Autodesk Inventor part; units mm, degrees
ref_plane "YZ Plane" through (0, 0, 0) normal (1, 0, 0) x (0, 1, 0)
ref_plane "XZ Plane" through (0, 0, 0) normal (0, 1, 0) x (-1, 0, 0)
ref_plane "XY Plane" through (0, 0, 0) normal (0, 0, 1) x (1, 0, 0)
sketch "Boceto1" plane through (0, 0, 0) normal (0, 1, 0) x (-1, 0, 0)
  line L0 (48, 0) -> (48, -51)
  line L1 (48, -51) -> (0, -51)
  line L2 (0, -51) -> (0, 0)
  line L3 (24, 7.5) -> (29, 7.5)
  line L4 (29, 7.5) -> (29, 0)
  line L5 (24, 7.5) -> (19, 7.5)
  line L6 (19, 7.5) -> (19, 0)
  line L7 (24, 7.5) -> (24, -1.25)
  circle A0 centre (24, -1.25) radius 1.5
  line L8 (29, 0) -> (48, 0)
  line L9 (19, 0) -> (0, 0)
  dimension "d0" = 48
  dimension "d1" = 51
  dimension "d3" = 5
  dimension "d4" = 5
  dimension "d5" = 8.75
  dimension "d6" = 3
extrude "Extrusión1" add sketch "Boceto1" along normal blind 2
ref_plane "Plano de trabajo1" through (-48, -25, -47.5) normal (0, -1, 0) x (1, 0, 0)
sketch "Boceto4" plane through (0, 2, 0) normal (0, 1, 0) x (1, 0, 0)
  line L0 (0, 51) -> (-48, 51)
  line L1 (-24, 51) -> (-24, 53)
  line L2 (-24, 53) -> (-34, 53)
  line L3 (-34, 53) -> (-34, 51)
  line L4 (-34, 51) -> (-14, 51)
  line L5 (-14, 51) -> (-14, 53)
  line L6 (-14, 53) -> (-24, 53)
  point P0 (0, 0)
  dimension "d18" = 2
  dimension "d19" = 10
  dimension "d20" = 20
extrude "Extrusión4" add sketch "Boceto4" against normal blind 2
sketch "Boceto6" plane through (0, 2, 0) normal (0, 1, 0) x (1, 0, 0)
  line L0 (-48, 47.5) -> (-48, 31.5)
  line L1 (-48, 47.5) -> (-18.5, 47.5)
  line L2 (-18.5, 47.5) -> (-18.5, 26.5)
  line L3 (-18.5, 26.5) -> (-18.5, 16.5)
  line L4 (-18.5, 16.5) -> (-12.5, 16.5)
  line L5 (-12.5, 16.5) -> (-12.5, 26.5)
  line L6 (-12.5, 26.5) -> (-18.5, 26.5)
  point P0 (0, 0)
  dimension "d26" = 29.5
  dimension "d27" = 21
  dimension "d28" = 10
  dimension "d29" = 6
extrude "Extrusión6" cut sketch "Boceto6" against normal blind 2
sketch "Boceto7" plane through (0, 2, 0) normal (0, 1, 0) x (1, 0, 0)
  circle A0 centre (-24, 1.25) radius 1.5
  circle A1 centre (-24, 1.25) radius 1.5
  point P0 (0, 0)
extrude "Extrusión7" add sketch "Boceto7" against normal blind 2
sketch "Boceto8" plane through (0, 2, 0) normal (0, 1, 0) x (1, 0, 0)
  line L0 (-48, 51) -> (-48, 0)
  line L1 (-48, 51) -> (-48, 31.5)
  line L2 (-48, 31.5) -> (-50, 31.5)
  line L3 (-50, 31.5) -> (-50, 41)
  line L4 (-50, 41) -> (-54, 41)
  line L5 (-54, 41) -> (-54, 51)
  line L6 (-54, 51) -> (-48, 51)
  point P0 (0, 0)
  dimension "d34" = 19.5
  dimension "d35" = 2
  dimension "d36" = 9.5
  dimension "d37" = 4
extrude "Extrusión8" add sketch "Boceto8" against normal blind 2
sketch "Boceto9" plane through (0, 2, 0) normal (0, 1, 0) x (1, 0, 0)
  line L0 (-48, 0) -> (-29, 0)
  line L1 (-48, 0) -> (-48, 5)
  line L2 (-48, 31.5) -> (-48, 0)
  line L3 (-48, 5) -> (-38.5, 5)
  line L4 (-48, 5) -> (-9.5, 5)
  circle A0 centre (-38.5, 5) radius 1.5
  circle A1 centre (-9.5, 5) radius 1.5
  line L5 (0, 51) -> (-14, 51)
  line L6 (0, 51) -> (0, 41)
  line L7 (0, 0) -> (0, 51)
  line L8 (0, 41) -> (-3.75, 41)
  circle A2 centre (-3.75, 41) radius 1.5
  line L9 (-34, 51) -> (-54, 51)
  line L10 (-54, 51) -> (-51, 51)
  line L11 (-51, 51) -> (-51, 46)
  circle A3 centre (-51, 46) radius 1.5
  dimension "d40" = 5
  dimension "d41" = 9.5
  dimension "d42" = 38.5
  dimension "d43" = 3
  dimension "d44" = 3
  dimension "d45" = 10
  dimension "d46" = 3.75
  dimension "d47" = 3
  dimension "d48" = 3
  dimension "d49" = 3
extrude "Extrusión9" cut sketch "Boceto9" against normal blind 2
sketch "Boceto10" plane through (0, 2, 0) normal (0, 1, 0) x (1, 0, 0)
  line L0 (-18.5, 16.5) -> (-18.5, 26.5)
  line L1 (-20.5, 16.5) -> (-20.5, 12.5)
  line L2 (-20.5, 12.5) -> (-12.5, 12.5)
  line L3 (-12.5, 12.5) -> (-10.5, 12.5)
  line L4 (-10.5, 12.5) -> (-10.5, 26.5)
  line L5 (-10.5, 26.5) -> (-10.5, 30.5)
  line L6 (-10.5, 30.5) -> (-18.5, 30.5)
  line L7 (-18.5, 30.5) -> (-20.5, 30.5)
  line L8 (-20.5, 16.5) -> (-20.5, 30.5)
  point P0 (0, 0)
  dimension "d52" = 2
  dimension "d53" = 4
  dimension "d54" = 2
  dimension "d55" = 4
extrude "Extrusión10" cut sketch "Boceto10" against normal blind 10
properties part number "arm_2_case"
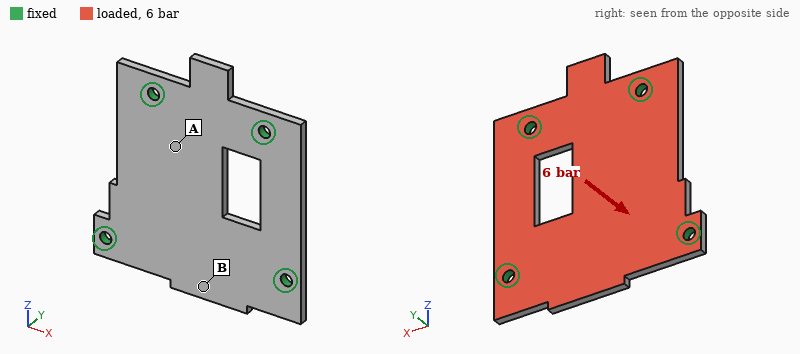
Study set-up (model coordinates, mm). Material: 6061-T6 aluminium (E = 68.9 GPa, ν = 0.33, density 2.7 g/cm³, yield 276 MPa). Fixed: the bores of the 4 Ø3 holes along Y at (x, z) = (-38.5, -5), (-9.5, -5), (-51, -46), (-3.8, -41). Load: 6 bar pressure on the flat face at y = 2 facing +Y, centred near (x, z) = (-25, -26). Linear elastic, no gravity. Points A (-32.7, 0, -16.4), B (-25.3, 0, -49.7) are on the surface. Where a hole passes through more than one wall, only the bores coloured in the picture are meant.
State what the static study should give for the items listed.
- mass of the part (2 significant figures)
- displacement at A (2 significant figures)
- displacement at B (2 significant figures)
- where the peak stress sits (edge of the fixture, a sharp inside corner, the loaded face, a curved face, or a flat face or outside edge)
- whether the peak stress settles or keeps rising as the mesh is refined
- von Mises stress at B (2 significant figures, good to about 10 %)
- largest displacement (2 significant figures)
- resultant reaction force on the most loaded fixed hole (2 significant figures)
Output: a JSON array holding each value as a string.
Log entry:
["13 g", "0.11 mm", "0.20 mm", "edge of the fixture", "keeps rising", "88 MPa", "0.21 mm", "420 N"]
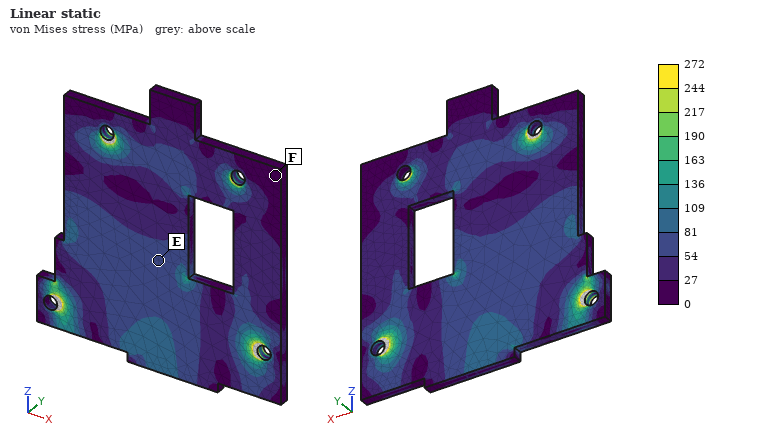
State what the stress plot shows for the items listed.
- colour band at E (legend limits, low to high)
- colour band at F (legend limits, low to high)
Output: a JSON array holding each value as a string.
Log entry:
["54 to 81 MPa", "0 to 27 MPa"]
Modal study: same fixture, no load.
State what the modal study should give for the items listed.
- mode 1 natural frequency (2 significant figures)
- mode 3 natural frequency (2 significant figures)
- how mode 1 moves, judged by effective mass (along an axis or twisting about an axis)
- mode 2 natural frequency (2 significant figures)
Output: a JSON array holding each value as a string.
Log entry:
["4200 Hz", "7700 Hz", "along Y", "5700 Hz"]
